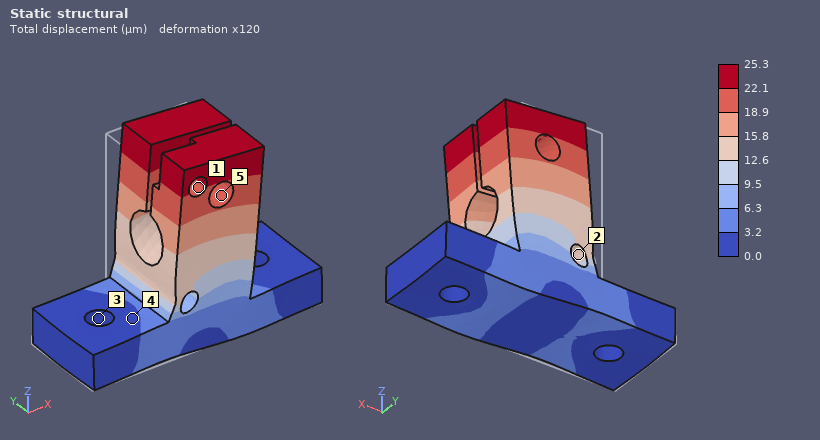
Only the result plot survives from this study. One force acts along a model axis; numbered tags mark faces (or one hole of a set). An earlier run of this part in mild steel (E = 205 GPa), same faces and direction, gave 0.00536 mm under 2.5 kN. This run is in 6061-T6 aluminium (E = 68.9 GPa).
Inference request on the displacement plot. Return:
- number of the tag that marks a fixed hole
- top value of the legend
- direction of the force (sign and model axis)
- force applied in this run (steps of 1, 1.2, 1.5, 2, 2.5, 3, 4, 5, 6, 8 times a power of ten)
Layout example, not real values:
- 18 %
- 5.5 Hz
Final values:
- 3
- 25.3 µm
- +X
- 4 kN
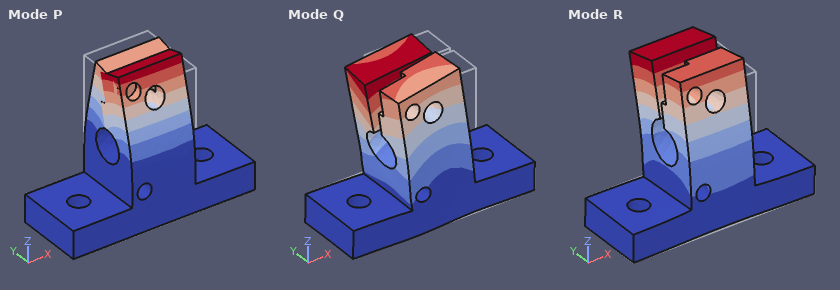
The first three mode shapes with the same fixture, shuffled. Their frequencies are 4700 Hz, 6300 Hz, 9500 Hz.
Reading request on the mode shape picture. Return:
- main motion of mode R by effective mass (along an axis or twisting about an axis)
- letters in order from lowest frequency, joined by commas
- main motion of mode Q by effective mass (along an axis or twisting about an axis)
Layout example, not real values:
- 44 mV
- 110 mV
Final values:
- along Y
- R, P, Q
- along X
